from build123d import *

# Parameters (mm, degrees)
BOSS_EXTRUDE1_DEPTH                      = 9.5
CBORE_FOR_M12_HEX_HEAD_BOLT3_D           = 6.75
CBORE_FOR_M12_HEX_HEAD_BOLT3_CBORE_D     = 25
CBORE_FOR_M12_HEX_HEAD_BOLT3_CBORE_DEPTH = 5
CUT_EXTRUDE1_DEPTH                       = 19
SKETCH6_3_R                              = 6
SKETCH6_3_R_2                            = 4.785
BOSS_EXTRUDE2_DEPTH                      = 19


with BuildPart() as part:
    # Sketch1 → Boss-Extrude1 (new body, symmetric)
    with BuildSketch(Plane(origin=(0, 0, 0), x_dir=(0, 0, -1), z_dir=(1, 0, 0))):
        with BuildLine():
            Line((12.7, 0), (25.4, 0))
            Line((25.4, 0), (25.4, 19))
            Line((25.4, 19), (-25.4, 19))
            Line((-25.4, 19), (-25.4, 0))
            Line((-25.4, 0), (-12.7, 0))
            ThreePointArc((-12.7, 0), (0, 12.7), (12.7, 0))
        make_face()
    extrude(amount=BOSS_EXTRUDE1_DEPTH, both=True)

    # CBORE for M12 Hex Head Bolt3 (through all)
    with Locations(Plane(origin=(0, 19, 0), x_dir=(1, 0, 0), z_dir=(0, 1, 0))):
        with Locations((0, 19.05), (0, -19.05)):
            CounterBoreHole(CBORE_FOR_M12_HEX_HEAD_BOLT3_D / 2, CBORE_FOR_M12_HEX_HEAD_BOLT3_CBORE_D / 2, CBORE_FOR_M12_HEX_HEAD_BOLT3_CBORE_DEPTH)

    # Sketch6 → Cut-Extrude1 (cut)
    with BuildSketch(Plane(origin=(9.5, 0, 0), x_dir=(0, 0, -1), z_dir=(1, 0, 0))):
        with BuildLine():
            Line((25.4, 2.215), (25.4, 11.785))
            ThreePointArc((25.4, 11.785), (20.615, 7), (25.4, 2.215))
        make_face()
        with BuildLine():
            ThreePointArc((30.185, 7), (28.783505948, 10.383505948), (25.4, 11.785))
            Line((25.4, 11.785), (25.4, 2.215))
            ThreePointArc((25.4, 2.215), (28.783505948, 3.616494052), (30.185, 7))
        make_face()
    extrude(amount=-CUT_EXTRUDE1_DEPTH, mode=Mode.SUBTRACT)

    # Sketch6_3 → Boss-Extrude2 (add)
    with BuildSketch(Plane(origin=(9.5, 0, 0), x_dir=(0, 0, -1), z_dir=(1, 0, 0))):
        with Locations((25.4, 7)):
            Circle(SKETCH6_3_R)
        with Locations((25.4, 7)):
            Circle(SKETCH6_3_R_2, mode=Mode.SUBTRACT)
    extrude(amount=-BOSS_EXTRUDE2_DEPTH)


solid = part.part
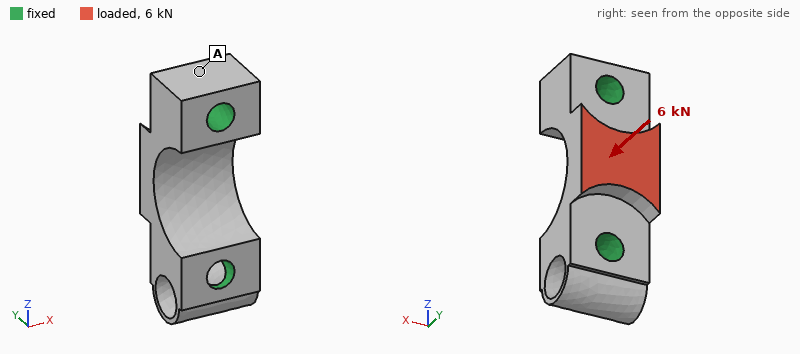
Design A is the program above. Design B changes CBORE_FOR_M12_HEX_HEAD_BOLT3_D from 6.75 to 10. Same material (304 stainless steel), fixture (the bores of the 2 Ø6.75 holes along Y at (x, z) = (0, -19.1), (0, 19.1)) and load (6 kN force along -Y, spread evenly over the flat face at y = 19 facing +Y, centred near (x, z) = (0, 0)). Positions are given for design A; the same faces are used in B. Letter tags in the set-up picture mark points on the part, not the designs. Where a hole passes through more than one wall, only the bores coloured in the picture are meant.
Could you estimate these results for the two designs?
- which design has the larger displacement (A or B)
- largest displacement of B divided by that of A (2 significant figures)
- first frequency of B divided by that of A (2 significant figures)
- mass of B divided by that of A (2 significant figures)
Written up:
A
0.90
1.2
0.89
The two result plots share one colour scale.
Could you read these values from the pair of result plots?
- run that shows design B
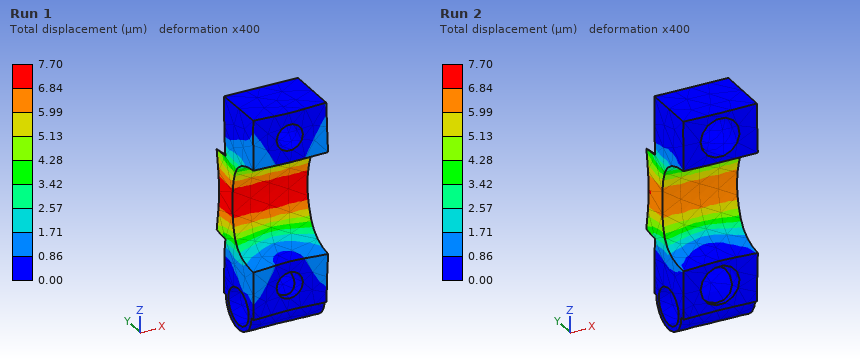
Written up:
Run 2
